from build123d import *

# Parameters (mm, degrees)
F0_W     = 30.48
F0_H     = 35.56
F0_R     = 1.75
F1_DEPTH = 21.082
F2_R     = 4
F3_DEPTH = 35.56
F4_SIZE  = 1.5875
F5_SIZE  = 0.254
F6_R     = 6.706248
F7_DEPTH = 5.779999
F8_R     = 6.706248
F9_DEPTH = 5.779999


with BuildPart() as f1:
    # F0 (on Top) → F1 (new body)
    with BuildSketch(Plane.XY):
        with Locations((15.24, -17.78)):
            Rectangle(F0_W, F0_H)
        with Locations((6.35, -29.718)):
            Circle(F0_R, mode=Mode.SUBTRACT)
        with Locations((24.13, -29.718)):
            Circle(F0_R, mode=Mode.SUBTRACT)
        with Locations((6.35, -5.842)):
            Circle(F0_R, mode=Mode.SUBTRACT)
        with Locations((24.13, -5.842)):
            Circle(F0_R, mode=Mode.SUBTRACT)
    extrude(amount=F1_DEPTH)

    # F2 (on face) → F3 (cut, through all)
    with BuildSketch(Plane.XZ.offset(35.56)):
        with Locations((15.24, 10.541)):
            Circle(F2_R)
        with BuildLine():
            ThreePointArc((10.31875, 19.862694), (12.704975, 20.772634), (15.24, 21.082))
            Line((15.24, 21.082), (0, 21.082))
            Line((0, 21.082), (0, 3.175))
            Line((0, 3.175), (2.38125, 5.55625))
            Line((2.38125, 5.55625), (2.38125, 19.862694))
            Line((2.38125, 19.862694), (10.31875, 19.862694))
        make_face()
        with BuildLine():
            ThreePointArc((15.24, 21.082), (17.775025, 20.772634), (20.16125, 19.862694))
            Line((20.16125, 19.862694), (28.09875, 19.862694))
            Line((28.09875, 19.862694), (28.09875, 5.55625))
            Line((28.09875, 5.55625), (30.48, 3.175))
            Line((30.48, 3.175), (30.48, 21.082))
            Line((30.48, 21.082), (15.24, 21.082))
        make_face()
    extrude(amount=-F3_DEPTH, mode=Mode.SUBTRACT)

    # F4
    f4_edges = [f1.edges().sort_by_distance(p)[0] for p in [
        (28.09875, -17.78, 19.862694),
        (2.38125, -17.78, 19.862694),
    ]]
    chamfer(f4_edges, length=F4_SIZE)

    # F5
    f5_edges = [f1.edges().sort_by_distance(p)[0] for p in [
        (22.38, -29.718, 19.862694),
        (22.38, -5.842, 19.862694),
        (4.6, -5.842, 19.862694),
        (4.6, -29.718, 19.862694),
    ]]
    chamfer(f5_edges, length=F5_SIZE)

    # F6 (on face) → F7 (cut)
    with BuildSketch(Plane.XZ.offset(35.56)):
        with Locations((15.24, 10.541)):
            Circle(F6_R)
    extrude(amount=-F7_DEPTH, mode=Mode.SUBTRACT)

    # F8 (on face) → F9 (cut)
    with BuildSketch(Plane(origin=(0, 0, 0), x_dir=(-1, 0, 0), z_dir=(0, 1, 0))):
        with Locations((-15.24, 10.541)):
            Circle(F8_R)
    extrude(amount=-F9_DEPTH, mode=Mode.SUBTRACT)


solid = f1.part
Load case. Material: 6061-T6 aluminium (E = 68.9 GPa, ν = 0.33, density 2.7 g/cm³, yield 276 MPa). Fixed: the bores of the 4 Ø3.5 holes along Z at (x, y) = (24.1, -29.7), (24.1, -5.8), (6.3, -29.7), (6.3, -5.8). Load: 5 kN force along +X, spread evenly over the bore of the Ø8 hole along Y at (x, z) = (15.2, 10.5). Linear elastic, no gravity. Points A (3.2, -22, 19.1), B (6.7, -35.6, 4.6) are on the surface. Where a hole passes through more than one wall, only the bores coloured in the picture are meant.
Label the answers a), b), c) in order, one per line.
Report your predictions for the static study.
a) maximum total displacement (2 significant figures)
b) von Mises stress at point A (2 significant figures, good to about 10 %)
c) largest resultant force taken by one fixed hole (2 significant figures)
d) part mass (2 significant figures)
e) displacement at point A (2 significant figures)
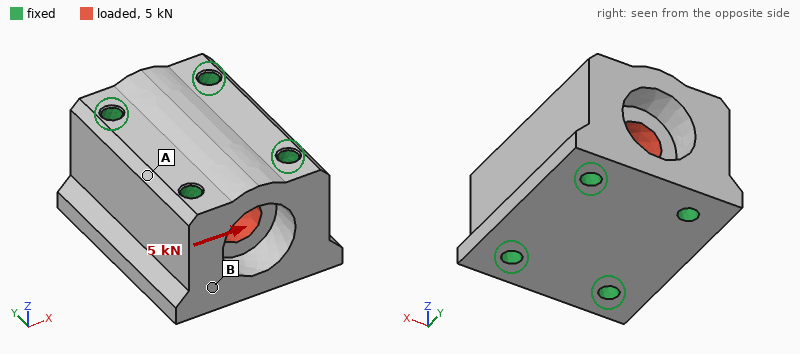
a) 2.1 µm
b) 4.0 MPa
c) 1.3 kN
d) 42 g
e) 1.3 µm
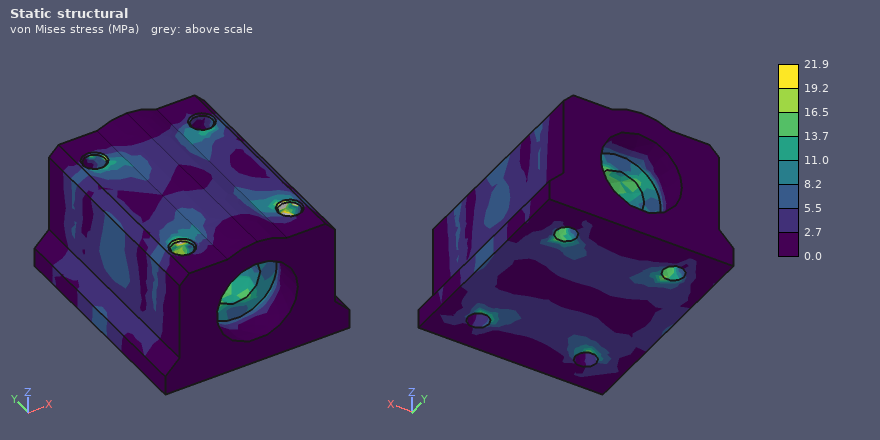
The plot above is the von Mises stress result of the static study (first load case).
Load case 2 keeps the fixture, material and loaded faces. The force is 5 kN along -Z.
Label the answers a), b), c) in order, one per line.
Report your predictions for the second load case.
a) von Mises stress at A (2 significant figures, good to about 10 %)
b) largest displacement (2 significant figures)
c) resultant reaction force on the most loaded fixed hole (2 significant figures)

a) 3.8 MPa
b) 3.0 µm
c) 1.3 kN
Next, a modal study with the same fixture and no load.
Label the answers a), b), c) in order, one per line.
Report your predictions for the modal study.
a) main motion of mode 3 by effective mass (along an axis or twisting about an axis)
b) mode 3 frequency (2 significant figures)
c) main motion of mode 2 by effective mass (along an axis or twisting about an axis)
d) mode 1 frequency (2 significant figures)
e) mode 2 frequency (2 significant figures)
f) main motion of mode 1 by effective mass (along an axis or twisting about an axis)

a) twisting about Y
b) 61 kHz
c) along X
d) 54 kHz
e) 57 kHz
f) along Z
